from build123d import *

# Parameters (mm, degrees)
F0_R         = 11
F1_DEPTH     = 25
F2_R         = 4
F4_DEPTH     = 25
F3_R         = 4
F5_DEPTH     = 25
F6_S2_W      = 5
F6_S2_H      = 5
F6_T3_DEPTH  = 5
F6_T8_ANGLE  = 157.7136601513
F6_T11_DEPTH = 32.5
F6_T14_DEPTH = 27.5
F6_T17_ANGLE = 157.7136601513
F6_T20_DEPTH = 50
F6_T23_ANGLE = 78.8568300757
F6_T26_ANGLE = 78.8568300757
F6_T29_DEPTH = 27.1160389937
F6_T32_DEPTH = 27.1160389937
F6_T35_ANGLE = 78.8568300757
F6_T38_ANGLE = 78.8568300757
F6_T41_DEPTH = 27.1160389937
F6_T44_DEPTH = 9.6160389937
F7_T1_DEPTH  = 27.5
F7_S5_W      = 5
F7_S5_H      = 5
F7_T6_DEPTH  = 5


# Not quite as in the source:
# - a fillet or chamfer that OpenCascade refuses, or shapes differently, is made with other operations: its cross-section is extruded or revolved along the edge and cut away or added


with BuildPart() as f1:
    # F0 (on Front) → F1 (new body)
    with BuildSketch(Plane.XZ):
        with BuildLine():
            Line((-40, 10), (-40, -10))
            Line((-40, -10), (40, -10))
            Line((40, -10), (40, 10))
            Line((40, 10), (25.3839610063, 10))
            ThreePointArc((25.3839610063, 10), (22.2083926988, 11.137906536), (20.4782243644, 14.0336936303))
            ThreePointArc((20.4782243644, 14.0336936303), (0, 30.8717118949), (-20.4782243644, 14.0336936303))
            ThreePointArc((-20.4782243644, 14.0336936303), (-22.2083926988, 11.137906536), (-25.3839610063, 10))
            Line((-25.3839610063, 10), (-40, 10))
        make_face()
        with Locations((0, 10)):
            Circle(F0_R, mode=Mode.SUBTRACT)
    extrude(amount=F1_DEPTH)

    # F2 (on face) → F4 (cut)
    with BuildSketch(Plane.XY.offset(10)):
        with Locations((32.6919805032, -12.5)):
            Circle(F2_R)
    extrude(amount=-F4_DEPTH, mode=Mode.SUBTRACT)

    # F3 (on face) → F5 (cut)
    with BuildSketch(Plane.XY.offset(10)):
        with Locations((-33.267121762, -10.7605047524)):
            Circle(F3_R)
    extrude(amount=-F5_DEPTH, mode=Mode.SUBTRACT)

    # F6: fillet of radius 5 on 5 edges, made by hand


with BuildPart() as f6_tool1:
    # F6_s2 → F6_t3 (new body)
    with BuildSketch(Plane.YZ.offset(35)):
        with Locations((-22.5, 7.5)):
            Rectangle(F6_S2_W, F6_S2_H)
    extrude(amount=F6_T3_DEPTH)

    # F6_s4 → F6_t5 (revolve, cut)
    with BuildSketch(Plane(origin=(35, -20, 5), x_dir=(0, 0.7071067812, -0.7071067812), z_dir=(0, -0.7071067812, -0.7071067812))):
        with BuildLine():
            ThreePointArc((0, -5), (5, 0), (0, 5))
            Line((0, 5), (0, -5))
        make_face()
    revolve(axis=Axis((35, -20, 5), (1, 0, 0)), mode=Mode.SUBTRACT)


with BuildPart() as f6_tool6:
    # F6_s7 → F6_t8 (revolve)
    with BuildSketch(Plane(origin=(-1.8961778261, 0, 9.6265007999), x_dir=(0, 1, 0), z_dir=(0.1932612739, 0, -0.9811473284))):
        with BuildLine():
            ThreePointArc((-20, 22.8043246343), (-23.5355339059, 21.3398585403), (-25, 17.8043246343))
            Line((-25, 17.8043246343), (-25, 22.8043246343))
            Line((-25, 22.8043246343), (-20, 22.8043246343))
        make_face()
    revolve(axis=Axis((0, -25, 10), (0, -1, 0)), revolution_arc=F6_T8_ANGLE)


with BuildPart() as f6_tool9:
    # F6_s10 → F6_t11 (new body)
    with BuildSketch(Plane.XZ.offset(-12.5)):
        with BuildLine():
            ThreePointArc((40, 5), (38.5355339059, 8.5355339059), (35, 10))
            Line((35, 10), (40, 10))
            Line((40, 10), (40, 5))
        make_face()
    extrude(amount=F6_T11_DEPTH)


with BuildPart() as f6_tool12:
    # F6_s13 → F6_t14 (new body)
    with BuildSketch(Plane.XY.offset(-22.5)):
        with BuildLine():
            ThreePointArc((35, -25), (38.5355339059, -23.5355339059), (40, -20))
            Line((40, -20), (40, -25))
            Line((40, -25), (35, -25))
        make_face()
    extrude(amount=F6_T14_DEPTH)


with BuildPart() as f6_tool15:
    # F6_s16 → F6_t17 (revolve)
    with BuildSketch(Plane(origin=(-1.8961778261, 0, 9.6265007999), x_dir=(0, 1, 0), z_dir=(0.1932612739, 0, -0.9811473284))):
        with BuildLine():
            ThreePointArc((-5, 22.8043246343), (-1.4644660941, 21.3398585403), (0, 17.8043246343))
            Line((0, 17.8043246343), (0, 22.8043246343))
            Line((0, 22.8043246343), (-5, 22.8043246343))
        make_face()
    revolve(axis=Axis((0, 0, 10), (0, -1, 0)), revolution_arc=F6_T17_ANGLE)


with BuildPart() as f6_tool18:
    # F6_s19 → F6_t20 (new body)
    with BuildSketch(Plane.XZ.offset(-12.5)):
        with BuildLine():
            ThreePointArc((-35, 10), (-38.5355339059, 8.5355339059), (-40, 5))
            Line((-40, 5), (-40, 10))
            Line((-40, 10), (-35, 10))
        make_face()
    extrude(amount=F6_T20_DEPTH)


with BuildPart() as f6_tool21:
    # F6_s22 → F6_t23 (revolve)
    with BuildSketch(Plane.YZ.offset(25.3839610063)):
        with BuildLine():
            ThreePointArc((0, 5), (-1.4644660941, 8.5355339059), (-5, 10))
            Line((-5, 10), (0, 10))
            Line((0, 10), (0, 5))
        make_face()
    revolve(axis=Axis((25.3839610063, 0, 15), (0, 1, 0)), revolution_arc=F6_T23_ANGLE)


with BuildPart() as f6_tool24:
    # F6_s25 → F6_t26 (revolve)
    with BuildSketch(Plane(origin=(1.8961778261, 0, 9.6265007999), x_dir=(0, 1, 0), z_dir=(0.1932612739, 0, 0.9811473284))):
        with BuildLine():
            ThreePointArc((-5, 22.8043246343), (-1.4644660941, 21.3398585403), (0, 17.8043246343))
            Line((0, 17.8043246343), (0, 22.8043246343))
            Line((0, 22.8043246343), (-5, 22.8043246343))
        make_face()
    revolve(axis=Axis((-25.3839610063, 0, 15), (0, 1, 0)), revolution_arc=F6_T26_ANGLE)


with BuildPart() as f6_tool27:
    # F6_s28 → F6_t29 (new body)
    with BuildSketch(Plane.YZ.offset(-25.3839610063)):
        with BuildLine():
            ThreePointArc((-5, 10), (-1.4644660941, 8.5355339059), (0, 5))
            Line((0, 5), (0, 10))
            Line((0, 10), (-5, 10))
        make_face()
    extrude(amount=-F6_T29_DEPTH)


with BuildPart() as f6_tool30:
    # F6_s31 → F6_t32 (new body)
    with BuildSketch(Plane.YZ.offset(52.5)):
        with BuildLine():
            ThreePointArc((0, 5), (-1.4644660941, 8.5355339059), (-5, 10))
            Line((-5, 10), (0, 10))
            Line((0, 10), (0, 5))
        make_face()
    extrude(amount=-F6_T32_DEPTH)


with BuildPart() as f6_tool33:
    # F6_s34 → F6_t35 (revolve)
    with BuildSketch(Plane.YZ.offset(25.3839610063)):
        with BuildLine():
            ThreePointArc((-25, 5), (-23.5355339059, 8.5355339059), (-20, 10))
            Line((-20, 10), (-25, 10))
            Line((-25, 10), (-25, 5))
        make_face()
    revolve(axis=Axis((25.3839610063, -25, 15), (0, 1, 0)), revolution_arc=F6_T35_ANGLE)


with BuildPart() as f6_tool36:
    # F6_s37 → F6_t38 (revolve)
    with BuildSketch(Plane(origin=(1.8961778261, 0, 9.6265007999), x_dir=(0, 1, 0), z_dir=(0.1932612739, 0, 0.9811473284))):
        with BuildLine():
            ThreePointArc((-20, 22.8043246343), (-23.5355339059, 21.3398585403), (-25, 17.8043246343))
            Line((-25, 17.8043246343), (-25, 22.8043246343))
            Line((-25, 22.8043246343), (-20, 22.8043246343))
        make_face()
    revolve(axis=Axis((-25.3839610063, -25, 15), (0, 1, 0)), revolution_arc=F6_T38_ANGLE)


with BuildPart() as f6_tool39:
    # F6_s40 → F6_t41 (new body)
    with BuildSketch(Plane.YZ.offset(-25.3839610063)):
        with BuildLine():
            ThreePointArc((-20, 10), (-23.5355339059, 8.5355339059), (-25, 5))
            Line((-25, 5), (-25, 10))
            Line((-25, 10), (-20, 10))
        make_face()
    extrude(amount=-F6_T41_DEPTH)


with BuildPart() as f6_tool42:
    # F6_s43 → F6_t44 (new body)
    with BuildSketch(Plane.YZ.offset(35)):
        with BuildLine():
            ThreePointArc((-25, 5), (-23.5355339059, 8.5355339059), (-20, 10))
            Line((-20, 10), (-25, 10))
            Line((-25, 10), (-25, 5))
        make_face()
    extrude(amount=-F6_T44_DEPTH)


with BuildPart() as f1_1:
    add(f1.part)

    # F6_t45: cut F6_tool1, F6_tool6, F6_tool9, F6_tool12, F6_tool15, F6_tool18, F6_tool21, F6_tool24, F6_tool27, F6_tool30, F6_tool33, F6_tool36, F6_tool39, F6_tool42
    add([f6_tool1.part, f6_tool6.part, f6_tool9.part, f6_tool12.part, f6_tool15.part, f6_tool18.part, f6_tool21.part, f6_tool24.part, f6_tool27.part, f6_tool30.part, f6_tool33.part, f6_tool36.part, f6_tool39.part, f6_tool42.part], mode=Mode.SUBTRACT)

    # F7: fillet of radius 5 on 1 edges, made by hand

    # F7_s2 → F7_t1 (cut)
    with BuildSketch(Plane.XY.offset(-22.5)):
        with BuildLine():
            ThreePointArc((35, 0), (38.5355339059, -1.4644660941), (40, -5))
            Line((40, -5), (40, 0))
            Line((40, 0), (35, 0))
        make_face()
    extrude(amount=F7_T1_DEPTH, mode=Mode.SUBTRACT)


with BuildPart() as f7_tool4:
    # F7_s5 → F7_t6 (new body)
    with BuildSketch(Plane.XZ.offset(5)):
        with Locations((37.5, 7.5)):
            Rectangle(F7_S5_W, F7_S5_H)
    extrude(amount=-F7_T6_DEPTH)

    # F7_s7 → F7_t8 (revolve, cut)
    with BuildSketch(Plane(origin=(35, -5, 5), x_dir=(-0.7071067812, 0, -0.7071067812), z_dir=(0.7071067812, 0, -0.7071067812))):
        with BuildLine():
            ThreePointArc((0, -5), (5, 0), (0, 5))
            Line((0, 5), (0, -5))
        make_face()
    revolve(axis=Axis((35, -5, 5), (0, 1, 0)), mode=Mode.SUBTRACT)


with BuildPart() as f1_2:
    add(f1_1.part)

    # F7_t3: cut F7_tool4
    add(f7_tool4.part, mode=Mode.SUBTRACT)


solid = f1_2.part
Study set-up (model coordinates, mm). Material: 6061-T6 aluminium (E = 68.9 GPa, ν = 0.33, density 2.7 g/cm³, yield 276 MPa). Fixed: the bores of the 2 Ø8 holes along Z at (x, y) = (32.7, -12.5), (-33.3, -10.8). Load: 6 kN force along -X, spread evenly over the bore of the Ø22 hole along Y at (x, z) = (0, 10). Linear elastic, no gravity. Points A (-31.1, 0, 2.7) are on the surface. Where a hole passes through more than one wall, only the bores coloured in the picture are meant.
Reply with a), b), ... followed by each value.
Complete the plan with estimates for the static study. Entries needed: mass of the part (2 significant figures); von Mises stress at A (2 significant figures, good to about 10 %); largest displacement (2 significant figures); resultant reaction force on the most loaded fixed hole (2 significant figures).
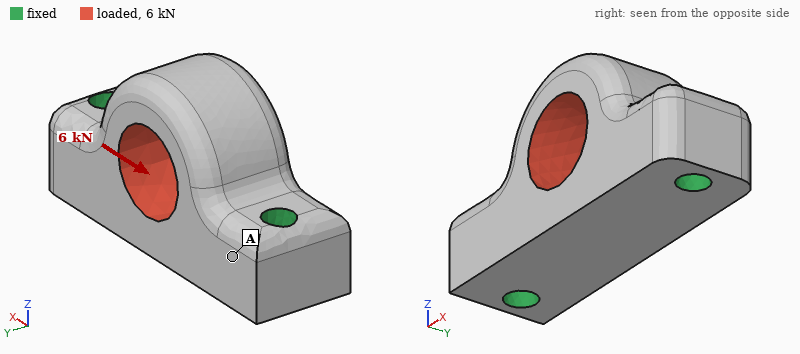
a) 120 g
b) 3.6 MPa
c) 8.0 µm
d) 3.1 kN
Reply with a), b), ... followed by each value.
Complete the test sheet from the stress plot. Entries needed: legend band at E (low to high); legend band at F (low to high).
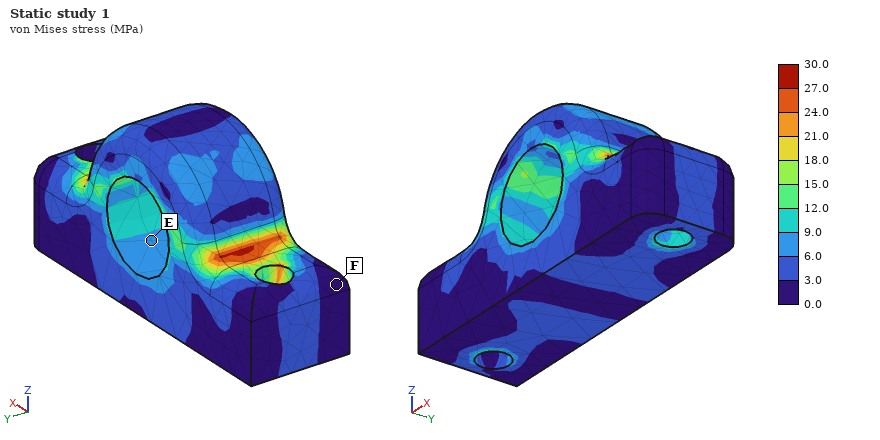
a) 6.0 to 9.0 MPa
b) 0.0 to 3.0 MPa
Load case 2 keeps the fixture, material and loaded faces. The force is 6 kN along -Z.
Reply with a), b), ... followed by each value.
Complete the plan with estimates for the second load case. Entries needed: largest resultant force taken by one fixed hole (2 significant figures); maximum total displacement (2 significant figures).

a) 3.0 kN
b) 11 µm
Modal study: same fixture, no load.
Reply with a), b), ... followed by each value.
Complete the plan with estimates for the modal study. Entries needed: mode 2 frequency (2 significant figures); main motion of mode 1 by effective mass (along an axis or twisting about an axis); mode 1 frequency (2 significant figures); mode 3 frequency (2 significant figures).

a) 16 kHz
b) along Y
c) 9700 Hz
d) 17 kHz
